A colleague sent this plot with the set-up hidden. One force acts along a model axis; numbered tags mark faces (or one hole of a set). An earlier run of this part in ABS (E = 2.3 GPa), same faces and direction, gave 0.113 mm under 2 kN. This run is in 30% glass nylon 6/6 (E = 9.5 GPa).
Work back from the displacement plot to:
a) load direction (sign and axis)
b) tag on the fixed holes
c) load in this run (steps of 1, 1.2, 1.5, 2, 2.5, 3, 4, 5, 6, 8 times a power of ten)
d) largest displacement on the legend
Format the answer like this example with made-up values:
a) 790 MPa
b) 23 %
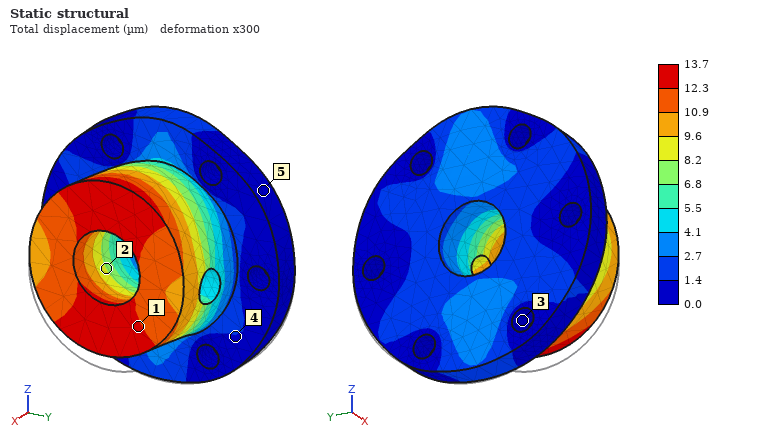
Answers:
a) +Z
b) 3
c) 1 kN
d) 13.7 µm
